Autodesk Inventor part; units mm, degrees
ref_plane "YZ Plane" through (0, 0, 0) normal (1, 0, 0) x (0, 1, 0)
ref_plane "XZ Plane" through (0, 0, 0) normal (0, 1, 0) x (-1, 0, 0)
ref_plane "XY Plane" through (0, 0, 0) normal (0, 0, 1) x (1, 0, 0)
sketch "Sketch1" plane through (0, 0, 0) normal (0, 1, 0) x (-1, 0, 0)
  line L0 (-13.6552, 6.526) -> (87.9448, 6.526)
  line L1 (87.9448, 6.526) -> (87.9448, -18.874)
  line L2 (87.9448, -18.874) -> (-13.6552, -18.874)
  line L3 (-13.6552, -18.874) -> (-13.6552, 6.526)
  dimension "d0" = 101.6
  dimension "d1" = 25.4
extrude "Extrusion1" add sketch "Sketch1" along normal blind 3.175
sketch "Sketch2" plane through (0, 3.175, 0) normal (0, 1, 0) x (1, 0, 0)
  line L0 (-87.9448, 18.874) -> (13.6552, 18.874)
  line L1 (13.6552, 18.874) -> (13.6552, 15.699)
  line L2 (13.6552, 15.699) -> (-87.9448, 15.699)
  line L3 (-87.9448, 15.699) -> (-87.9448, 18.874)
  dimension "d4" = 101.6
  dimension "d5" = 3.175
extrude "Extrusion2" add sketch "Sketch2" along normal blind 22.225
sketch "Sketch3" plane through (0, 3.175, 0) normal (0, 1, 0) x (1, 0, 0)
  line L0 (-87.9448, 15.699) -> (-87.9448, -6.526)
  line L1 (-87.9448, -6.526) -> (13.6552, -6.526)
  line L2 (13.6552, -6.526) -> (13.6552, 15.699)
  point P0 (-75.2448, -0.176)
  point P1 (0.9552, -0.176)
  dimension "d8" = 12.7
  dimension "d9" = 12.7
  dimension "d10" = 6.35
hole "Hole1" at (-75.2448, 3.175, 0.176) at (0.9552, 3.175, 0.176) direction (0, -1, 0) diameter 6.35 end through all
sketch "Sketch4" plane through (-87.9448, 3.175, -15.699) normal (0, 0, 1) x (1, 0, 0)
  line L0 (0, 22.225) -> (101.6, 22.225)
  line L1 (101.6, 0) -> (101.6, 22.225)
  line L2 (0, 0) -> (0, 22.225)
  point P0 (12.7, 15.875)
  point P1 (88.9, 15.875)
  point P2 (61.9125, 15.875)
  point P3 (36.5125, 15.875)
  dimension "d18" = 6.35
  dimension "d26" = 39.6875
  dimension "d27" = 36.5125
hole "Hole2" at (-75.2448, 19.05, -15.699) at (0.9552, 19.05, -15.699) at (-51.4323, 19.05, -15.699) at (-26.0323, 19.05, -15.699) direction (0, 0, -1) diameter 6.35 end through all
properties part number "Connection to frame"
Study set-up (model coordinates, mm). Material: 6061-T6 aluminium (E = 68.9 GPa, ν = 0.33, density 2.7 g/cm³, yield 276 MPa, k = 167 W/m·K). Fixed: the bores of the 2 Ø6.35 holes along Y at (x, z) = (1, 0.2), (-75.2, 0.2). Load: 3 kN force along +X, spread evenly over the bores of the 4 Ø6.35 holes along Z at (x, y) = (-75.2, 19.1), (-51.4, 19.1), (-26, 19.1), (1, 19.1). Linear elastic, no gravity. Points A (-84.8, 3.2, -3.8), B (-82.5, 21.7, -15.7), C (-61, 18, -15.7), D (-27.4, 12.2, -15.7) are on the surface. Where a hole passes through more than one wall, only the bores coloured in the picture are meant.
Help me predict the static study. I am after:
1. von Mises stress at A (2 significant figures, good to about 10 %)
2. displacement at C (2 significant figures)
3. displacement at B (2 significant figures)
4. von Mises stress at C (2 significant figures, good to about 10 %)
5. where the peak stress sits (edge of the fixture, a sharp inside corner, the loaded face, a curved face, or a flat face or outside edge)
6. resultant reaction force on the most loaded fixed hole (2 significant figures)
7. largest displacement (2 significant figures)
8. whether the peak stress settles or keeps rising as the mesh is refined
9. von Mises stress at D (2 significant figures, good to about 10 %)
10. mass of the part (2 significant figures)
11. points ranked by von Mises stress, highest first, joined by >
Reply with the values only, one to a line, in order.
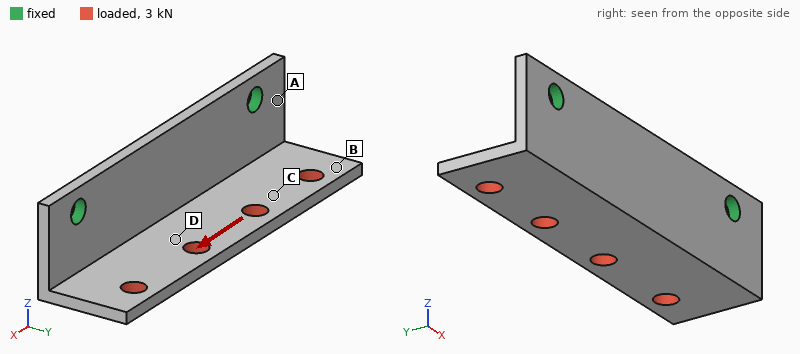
93 MPa
0.14 mm
0.26 mm
41 MPa
edge of the fixture
1.7 kN
0.32 mm
keeps rising
60 MPa
40 g
A > D > C > B
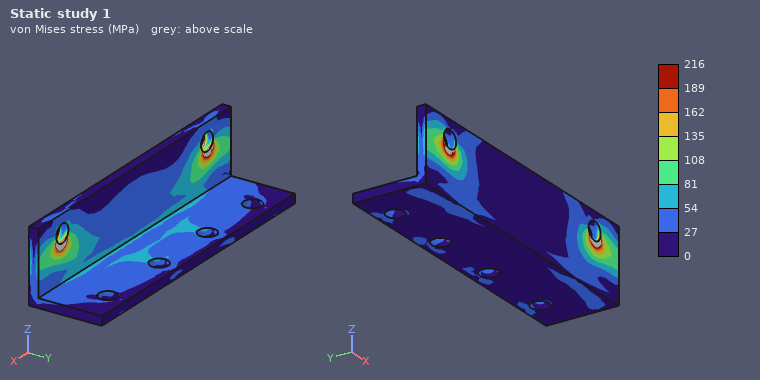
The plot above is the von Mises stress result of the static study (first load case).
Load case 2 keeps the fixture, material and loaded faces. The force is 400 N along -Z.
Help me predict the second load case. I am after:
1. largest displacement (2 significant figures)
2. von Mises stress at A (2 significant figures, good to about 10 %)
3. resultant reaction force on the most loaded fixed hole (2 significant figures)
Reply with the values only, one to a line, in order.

0.27 mm
43 MPa
220 N
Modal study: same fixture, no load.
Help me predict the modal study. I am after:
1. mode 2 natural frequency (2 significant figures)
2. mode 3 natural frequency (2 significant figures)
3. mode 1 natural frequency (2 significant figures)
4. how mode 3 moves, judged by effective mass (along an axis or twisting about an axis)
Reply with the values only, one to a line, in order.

2900 Hz
3900 Hz
1800 Hz
along Y
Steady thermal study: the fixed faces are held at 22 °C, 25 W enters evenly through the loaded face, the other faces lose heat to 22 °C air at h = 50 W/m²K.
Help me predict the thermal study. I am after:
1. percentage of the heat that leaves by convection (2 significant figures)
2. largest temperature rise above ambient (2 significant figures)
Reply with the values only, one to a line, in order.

23 %
21 K
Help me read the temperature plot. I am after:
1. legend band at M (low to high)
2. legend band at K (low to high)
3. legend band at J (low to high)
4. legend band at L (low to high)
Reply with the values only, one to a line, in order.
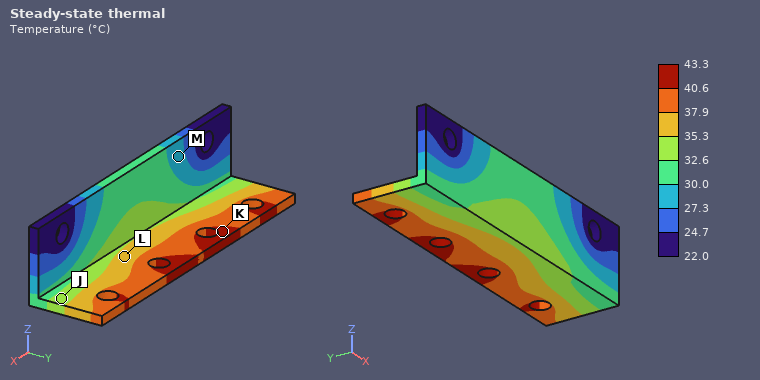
27.3 to 30.0 °C
40.6 to 43.3 °C
32.6 to 35.3 °C
35.3 to 37.9 °C
